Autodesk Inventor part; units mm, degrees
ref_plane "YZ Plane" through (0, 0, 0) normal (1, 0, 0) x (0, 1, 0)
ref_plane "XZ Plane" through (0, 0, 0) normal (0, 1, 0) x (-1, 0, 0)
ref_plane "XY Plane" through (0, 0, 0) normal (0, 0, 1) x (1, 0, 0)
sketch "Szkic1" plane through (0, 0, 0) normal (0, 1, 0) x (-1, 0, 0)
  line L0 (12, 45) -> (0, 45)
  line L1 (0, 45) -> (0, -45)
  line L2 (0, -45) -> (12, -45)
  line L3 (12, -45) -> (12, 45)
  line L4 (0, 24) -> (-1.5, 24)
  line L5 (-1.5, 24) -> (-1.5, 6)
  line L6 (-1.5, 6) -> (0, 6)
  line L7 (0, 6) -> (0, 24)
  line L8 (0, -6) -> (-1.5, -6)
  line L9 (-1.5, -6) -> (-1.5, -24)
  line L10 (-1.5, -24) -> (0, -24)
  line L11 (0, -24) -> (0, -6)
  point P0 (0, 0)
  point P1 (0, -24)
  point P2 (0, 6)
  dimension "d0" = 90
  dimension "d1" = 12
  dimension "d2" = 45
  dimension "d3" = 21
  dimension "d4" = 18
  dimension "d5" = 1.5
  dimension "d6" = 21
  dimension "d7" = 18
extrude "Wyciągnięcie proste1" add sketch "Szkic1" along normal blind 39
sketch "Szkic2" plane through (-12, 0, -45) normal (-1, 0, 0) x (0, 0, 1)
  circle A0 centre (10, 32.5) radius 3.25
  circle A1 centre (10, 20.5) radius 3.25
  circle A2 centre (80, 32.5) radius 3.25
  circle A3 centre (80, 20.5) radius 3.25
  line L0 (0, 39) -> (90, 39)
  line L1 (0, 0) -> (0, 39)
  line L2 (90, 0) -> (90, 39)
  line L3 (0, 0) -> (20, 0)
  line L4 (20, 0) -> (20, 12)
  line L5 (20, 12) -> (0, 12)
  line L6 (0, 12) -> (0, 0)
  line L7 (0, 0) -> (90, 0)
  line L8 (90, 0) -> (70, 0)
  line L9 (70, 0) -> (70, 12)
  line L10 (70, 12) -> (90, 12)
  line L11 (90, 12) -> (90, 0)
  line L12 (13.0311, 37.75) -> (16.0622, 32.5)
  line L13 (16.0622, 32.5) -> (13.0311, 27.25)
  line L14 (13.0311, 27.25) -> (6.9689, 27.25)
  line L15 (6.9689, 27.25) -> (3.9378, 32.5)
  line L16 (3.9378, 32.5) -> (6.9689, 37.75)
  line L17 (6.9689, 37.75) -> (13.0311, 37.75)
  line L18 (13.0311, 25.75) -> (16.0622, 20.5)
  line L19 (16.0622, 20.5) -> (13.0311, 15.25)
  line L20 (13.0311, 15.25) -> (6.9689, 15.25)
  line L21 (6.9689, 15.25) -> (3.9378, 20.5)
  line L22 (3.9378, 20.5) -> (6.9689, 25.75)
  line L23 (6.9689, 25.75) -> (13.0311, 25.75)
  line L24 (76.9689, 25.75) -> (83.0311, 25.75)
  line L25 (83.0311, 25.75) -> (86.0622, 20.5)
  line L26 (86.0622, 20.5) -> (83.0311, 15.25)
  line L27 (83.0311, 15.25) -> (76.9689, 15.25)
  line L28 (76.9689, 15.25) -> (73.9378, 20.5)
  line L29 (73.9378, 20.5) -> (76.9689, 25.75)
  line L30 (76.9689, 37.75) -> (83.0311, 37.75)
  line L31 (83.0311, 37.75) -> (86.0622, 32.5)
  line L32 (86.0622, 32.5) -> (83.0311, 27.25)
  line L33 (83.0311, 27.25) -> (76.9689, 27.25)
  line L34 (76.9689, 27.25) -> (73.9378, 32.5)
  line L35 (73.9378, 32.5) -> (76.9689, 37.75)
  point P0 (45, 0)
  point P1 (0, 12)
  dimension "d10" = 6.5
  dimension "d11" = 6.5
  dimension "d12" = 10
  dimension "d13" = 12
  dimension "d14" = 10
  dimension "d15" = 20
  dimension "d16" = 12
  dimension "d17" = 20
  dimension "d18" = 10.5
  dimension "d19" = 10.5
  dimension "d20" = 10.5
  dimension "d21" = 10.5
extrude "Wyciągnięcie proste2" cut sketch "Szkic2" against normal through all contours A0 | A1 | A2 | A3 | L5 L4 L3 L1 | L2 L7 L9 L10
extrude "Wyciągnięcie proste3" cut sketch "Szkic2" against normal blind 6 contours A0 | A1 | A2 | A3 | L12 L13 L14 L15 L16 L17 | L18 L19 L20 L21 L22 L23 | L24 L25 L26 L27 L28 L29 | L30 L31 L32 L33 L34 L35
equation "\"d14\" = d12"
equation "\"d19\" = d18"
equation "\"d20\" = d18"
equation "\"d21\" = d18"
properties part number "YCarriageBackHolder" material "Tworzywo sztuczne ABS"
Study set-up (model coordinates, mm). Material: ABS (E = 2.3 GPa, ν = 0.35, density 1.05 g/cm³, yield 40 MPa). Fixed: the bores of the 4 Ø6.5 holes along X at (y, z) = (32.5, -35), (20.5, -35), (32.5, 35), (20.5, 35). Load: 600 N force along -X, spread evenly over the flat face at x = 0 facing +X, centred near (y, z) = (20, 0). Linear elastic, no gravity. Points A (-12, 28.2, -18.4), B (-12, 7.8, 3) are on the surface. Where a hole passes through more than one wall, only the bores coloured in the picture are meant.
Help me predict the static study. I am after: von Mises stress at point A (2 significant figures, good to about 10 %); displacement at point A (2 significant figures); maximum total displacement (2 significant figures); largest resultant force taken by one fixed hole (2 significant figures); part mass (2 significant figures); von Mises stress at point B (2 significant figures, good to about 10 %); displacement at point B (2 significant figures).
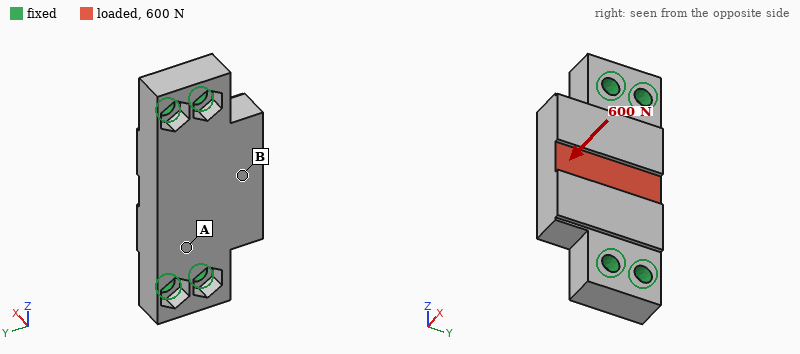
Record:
2.4 MPa
0.088 mm
0.27 mm
320 N
37 g
6.1 MPa
0.22 mm
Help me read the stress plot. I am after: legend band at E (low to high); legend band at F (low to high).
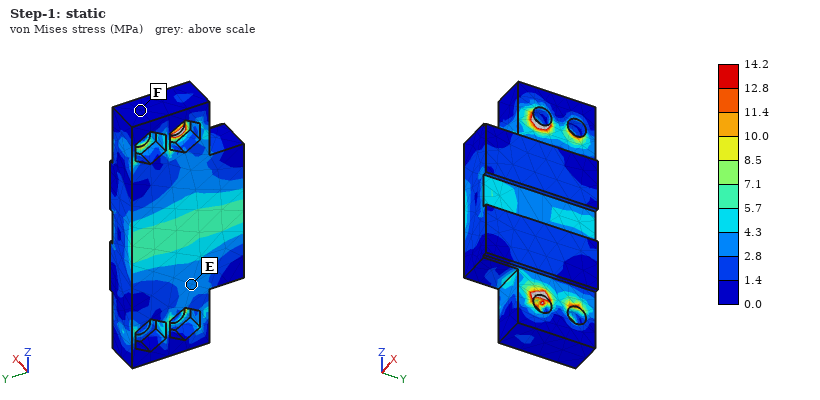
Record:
2.8 to 4.3 MPa
0.0 to 1.4 MPa
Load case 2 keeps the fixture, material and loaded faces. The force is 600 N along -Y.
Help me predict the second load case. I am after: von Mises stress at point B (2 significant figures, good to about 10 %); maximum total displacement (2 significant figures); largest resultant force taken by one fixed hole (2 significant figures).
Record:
1.8 MPa
0.11 mm
210 N
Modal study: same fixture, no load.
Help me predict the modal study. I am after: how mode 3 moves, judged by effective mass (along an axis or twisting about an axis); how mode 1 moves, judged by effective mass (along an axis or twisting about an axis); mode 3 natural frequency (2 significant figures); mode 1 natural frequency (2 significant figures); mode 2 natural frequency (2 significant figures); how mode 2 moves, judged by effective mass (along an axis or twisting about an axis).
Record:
along Y
along X
4100 Hz
2000 Hz
3200 Hz
along X
